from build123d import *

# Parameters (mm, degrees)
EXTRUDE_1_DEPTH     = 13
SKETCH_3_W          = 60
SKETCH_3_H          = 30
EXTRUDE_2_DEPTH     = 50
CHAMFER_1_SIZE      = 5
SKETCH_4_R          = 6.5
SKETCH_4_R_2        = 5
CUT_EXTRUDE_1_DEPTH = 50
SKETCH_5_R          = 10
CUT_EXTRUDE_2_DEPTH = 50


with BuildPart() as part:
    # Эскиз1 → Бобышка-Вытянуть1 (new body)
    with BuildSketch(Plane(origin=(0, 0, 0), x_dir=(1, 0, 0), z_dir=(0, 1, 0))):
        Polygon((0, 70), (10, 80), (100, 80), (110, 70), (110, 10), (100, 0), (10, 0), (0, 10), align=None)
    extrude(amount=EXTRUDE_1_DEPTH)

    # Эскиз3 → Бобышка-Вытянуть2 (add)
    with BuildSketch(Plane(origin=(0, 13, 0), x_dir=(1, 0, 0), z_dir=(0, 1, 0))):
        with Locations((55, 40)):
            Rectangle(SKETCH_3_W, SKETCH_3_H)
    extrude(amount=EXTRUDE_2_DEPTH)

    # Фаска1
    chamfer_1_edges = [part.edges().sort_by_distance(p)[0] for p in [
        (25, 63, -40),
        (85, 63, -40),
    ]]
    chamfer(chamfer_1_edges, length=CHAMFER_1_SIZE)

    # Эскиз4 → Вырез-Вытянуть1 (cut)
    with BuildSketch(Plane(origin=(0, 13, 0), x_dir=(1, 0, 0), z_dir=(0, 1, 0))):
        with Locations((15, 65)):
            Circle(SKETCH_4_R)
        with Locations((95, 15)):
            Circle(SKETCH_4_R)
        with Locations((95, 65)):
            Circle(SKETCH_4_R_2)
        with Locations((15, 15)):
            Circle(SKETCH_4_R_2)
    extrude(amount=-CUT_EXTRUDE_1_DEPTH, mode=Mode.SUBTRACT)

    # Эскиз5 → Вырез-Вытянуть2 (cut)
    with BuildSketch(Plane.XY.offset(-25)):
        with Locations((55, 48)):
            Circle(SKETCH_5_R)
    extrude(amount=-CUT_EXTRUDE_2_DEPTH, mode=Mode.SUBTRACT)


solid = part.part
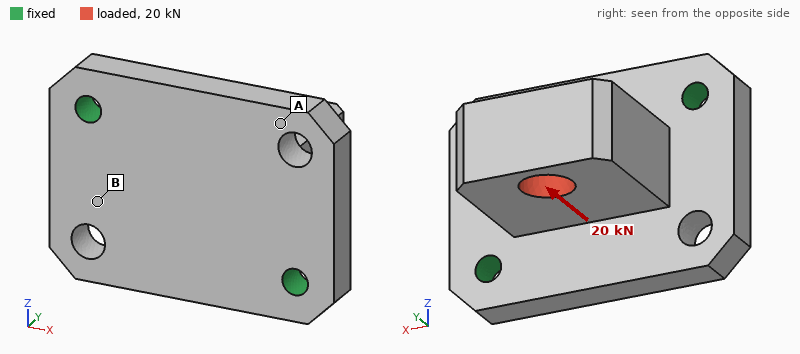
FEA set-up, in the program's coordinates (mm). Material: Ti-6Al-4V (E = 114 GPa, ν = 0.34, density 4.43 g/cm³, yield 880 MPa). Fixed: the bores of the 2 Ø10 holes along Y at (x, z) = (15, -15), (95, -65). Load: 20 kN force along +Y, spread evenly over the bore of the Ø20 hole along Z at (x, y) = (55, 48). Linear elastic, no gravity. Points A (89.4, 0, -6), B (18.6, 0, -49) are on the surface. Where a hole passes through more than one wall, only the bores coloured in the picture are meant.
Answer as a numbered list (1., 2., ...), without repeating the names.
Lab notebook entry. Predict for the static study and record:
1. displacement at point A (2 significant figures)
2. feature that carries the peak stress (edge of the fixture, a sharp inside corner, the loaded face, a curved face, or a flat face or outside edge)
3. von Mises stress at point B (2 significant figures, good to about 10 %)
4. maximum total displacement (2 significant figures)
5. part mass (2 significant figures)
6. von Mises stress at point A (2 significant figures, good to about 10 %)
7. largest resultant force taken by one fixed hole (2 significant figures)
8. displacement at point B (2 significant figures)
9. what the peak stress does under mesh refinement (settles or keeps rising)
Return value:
1. 41 µm
2. edge of the fixture
3. 26 MPa
4. 44 µm
5. 820 g
6. 13 MPa
7. 11 kN
8. 30 µm
9. keeps rising
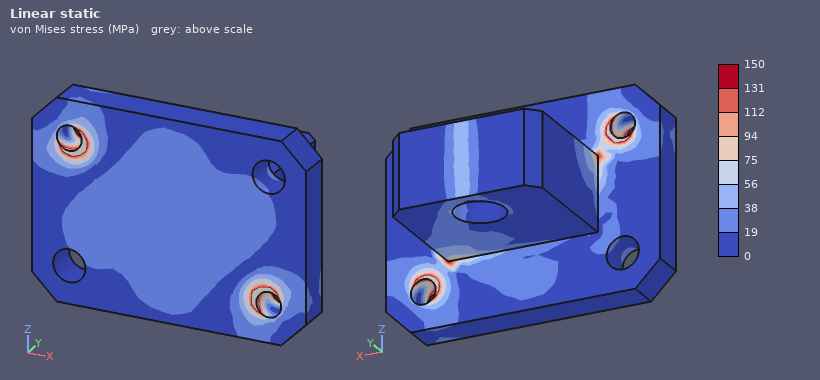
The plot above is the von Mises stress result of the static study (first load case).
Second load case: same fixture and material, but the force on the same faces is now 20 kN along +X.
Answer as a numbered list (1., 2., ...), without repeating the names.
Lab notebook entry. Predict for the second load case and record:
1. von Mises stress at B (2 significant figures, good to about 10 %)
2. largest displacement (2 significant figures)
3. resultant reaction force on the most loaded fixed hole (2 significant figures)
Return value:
1. 61 MPa
2. 0.24 mm
3. 13 kN
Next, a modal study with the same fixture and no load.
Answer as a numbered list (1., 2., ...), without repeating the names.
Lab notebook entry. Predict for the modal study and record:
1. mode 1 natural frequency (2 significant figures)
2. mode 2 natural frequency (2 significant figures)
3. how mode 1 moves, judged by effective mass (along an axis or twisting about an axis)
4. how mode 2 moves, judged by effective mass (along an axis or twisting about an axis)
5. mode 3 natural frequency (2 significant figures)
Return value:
1. 2000 Hz
2. 4400 Hz
3. along Z
4. along Y
5. 5600 Hz
